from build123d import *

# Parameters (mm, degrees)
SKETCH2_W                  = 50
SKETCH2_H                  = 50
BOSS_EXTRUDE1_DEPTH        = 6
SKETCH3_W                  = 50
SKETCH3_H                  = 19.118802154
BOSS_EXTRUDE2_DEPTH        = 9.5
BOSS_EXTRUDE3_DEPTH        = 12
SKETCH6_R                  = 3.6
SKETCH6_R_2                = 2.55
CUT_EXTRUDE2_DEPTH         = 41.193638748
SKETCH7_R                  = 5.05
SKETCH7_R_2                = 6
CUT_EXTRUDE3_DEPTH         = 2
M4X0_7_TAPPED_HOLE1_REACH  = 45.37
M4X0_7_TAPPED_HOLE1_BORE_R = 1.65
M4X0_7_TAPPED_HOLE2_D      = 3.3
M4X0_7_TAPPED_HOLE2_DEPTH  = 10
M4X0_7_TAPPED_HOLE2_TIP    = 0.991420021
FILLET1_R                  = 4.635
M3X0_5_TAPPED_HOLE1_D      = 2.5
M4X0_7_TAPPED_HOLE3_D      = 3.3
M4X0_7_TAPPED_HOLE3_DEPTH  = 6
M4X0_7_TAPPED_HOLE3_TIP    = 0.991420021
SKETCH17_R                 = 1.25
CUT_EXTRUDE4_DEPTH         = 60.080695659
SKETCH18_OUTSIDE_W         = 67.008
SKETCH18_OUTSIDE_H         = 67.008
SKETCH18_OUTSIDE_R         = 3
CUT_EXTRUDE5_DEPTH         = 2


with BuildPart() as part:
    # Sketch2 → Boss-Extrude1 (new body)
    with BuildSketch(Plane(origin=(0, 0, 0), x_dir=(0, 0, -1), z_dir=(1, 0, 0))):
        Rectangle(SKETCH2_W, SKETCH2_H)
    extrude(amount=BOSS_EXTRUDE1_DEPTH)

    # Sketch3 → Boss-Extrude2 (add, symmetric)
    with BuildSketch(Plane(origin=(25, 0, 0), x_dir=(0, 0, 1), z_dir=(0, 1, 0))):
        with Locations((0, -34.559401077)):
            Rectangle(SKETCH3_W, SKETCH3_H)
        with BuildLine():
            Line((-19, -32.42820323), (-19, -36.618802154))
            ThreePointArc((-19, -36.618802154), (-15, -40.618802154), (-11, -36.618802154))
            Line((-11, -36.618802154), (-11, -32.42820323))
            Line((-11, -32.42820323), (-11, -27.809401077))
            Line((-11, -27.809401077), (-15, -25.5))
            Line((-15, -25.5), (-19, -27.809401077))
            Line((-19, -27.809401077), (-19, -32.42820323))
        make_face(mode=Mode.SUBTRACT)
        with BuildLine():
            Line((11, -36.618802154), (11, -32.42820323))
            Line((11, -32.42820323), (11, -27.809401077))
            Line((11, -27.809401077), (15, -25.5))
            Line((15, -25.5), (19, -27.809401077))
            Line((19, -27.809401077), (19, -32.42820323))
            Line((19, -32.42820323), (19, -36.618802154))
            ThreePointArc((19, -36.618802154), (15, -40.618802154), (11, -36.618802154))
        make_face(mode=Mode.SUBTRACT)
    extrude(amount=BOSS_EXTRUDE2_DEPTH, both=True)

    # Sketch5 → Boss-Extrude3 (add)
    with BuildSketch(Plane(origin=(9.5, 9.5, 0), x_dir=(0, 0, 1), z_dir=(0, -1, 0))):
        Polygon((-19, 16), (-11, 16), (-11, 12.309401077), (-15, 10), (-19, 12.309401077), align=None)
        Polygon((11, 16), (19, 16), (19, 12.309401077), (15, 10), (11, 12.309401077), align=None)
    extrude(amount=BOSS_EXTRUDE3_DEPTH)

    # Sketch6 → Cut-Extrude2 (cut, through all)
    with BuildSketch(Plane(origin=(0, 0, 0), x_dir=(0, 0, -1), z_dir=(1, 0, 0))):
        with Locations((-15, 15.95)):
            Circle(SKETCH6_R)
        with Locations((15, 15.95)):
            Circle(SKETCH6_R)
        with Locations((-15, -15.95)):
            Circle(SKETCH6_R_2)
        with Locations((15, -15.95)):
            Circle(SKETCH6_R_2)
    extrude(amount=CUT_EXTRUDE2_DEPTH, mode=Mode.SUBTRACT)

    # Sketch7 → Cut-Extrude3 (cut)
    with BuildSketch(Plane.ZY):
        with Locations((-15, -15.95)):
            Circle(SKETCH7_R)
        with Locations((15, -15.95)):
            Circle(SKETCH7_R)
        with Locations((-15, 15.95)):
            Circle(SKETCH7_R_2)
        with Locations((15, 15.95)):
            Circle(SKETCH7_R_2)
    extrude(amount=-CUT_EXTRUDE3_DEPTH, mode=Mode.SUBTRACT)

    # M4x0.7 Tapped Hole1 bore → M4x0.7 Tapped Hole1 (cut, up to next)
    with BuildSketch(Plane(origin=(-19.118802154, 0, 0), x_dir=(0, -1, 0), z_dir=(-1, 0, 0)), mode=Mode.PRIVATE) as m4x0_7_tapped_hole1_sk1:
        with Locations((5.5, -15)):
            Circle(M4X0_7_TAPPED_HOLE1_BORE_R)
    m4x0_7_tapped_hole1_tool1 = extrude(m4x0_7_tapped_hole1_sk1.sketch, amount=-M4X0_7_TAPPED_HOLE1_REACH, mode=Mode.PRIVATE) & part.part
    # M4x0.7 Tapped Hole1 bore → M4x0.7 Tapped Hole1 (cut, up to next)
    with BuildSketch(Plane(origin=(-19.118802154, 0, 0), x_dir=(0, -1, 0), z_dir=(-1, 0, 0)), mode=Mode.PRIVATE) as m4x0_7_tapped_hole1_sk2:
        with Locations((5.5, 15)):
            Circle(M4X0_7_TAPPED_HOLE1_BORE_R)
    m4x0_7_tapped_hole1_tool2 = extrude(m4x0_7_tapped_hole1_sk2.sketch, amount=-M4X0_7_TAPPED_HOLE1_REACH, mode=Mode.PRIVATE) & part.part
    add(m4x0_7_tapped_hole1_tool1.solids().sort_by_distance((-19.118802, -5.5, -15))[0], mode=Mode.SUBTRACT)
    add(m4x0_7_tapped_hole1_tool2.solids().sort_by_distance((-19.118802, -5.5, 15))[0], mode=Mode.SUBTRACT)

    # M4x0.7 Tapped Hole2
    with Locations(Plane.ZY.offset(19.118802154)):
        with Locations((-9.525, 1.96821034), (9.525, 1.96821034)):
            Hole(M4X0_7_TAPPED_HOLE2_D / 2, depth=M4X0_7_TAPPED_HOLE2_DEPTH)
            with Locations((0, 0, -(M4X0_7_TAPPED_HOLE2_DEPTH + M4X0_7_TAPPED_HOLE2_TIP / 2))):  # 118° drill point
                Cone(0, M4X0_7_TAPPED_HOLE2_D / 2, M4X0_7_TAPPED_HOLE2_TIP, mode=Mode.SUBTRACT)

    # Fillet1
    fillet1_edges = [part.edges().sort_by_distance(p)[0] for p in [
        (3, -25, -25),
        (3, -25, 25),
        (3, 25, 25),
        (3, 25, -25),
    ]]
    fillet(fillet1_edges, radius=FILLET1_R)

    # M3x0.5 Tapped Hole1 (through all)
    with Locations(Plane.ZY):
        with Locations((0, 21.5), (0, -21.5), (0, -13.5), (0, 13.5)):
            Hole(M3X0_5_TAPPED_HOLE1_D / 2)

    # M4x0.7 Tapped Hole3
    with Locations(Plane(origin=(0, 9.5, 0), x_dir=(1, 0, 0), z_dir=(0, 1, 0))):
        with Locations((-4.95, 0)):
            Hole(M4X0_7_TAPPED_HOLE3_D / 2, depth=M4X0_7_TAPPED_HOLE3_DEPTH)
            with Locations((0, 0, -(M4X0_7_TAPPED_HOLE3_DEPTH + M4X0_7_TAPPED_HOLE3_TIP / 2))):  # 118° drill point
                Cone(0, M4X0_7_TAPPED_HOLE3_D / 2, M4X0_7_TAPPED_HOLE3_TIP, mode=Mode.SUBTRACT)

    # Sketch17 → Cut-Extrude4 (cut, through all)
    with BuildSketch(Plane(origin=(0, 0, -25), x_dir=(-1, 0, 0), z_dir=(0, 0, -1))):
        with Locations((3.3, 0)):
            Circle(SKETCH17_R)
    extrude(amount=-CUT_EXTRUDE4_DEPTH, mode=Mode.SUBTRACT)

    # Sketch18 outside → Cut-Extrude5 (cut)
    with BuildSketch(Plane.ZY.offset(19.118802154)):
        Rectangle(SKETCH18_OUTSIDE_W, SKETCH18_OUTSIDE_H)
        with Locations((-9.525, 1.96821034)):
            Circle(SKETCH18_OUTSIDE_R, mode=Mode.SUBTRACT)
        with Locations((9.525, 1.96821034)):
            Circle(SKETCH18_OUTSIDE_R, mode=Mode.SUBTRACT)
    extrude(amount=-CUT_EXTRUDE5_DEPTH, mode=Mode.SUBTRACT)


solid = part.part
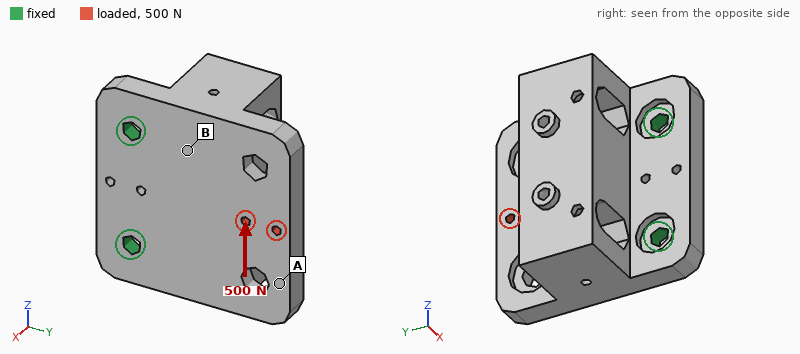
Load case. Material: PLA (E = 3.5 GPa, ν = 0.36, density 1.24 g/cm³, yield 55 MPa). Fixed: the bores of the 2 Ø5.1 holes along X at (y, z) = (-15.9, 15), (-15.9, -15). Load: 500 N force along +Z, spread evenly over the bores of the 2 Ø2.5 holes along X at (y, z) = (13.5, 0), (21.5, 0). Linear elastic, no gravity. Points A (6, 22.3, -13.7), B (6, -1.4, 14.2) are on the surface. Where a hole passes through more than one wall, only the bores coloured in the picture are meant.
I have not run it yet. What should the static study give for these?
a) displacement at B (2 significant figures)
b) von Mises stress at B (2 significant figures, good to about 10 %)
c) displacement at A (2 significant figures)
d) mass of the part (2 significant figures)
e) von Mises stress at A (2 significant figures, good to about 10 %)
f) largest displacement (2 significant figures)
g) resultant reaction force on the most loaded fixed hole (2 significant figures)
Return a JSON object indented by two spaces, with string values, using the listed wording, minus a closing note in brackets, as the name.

{
  "displacement at B": "0.049 mm",
  "von Mises stress at B": "4.7 MPa",
  "displacement at A": "0.12 mm",
  "mass of the part": "33 g",
  "von Mises stress at A": "2.4 MPa",
  "largest displacement": "0.13 mm",
  "resultant reaction force on the most loaded fixed hole": "570 N"
}
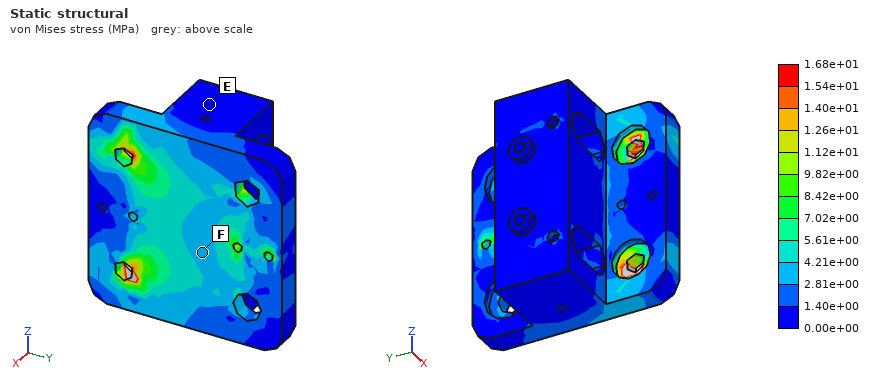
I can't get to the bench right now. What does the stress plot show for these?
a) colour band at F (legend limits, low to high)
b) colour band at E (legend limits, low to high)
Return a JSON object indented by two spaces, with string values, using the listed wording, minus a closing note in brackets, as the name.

{
  "colour band at F": "2.81e+00 to 4.21e+00 MPa",
  "colour band at E": "0.00e+00 to 1.40e+00 MPa"
}
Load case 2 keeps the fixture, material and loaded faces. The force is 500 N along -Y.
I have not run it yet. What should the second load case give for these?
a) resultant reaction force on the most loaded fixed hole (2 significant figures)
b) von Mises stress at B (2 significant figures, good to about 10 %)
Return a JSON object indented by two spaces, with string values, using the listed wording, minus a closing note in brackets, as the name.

{
  "resultant reaction force on the most loaded fixed hole": "260 N",
  "von Mises stress at B": "2.4 MPa"
}
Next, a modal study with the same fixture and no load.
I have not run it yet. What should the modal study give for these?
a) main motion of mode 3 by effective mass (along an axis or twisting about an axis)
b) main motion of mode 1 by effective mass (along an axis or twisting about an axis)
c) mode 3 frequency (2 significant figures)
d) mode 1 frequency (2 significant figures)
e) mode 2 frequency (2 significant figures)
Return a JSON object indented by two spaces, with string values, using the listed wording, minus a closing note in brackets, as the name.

{
  "main motion of mode 3 by effective mass": "along Z",
  "main motion of mode 1 by effective mass": "along X",
  "mode 3 frequency": "3200 Hz",
  "mode 1 frequency": "680 Hz",
  "mode 2 frequency": "2300 Hz"
}
